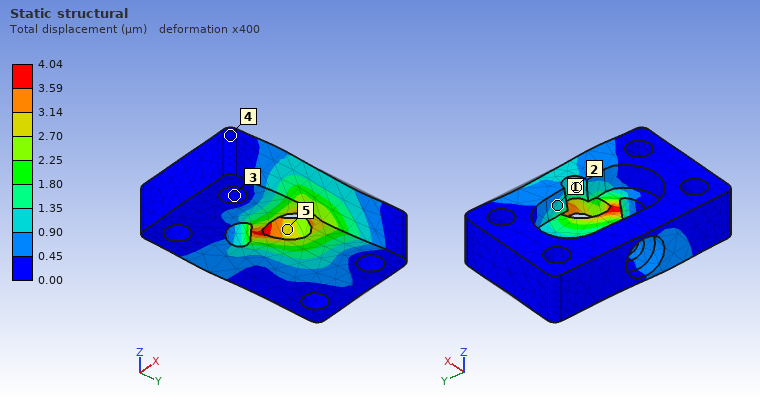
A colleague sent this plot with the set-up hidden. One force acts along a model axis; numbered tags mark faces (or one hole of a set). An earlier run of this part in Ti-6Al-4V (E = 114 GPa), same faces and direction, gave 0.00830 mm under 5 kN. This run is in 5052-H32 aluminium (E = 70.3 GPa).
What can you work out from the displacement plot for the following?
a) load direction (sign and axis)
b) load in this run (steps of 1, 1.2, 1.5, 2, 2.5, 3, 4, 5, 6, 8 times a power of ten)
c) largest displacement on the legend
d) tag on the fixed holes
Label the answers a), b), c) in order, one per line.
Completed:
a) -Y
b) 1.5 kN
c) 4.04 µm
d) 3
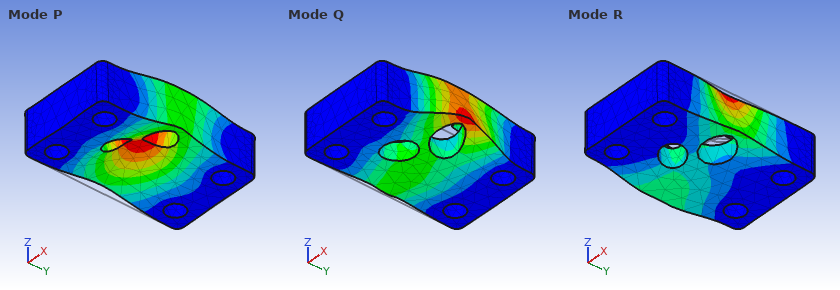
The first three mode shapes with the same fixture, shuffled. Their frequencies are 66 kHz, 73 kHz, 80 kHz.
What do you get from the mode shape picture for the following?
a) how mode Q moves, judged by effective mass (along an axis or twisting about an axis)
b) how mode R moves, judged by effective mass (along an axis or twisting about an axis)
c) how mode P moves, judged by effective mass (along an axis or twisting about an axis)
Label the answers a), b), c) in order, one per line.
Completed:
a) along X
b) along X
c) along Z
